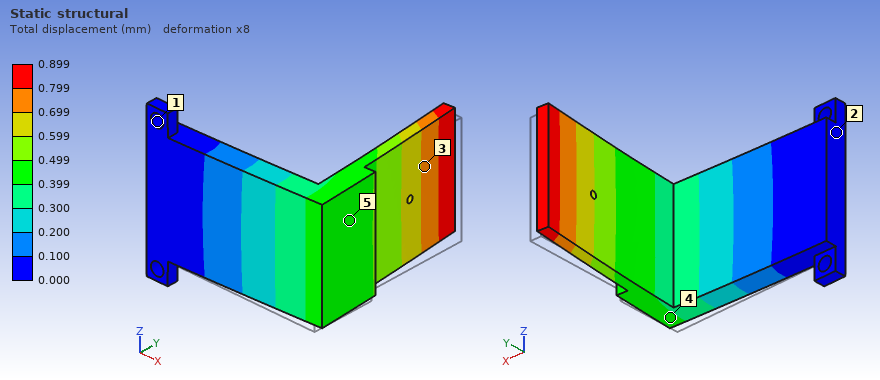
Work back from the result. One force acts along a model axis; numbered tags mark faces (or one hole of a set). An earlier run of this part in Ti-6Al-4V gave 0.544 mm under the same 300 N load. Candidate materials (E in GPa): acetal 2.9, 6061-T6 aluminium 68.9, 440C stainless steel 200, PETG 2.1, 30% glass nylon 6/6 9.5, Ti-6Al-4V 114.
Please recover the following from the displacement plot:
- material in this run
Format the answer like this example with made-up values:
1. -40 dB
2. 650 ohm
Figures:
1. 6061-T6 aluminium
